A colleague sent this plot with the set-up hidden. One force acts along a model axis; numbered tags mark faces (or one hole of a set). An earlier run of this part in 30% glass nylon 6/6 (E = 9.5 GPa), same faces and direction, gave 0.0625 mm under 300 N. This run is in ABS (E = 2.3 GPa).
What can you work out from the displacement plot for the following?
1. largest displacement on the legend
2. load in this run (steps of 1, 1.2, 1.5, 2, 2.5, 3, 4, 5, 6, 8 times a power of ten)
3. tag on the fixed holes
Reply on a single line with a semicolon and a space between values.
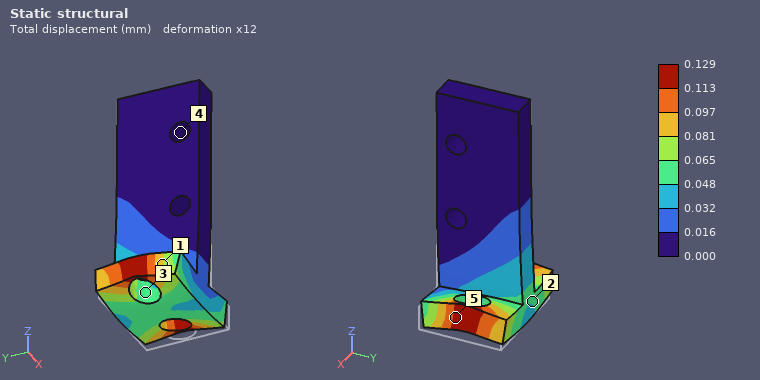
0.129 mm; 150 N; 4
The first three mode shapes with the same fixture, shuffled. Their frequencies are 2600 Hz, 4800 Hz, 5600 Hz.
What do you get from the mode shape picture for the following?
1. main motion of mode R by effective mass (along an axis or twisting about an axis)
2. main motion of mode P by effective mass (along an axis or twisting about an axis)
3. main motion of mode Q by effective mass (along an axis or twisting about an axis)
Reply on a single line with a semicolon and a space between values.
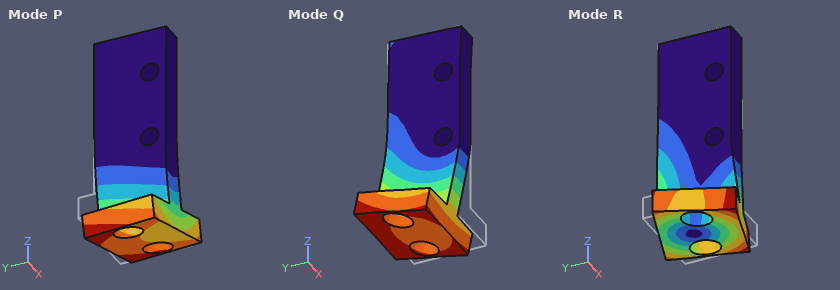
twisting about Z; along X; along Y
